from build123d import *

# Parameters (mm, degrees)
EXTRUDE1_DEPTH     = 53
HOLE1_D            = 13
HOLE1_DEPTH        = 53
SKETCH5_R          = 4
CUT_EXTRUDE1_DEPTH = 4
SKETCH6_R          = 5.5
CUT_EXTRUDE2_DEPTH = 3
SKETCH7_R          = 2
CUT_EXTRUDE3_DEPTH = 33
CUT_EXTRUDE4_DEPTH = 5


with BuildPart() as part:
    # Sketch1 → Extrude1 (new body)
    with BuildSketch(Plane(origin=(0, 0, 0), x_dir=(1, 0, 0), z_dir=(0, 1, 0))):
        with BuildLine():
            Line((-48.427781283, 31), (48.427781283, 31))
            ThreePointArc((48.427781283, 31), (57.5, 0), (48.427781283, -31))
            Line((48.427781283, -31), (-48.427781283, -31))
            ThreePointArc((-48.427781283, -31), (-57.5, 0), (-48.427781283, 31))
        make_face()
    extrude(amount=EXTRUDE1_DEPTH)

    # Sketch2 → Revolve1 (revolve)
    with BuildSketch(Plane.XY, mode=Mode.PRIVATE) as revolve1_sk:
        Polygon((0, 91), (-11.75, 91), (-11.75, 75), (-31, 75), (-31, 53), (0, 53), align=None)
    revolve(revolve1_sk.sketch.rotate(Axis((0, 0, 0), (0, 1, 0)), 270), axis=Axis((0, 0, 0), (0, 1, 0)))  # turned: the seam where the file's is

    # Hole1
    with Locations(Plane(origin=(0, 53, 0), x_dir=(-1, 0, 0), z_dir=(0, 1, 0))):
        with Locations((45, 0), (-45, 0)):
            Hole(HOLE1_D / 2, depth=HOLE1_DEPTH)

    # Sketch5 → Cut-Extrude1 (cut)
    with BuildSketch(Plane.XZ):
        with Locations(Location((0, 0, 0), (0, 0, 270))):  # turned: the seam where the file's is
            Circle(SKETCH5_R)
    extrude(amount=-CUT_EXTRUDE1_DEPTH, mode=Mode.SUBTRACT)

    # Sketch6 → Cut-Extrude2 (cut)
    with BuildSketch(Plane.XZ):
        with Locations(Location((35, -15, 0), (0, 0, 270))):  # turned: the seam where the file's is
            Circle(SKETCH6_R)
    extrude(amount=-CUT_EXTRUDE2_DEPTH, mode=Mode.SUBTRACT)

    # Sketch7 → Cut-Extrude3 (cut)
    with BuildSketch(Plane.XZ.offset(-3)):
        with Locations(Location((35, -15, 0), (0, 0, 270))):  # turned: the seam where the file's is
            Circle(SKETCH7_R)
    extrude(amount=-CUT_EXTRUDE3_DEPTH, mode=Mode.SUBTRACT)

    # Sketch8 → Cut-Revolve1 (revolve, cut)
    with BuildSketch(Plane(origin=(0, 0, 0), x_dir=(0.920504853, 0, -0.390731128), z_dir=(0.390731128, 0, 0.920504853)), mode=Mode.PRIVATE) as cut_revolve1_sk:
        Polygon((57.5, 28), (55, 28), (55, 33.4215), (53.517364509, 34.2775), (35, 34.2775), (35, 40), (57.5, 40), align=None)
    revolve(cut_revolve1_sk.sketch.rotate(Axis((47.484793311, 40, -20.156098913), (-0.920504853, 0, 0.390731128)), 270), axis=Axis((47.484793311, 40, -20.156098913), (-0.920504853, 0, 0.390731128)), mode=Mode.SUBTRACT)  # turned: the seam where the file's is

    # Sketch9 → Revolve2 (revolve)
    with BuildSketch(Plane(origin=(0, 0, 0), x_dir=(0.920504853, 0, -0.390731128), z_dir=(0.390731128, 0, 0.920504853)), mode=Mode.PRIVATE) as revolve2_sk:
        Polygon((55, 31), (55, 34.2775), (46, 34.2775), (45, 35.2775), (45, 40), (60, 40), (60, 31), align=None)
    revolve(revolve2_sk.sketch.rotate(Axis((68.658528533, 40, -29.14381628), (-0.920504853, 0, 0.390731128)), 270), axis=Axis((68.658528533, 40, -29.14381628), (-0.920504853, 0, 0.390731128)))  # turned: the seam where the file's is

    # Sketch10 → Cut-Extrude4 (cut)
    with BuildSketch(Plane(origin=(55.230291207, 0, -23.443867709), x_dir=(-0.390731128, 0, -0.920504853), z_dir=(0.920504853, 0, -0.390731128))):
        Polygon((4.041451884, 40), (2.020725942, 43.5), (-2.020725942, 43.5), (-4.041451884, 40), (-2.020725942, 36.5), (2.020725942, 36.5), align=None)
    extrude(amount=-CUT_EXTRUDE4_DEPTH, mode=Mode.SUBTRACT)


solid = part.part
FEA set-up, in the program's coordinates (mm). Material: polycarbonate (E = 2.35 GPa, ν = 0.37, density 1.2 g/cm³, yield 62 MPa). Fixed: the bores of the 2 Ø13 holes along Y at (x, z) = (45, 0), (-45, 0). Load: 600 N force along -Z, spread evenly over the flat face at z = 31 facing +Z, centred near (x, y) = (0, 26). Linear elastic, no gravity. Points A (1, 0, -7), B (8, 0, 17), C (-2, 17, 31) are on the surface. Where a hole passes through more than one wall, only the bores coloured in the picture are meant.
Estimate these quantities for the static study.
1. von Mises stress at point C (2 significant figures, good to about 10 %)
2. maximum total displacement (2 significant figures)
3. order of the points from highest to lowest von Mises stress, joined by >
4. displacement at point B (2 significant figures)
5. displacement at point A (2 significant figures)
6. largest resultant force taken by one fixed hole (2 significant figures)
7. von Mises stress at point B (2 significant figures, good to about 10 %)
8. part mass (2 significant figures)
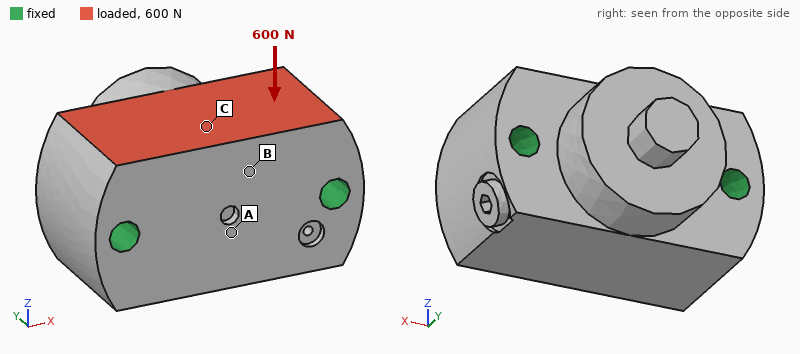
0.15 MPa
4.9 µm
C > B > A
4.2 µm
3.5 µm
310 N
0.097 MPa
500 g
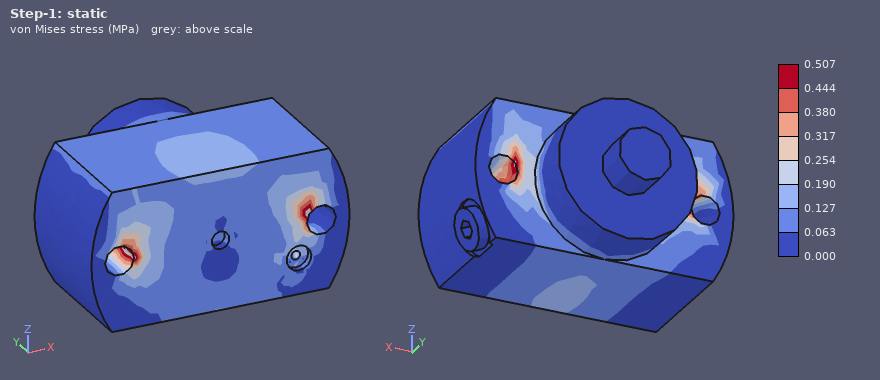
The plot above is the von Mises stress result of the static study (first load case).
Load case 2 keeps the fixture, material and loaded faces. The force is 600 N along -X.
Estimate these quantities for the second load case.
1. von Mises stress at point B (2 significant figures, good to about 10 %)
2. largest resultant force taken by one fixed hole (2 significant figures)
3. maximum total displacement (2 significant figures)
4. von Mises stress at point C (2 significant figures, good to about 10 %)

0.20 MPa
350 N
5.2 µm
0.20 MPa
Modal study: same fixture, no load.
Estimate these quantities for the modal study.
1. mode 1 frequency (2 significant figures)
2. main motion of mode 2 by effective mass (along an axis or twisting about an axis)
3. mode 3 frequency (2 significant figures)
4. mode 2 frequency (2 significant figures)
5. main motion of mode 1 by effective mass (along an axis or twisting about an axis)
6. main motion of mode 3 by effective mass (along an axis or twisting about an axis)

2200 Hz
along Y
3500 Hz
3200 Hz
along Z
along Z
